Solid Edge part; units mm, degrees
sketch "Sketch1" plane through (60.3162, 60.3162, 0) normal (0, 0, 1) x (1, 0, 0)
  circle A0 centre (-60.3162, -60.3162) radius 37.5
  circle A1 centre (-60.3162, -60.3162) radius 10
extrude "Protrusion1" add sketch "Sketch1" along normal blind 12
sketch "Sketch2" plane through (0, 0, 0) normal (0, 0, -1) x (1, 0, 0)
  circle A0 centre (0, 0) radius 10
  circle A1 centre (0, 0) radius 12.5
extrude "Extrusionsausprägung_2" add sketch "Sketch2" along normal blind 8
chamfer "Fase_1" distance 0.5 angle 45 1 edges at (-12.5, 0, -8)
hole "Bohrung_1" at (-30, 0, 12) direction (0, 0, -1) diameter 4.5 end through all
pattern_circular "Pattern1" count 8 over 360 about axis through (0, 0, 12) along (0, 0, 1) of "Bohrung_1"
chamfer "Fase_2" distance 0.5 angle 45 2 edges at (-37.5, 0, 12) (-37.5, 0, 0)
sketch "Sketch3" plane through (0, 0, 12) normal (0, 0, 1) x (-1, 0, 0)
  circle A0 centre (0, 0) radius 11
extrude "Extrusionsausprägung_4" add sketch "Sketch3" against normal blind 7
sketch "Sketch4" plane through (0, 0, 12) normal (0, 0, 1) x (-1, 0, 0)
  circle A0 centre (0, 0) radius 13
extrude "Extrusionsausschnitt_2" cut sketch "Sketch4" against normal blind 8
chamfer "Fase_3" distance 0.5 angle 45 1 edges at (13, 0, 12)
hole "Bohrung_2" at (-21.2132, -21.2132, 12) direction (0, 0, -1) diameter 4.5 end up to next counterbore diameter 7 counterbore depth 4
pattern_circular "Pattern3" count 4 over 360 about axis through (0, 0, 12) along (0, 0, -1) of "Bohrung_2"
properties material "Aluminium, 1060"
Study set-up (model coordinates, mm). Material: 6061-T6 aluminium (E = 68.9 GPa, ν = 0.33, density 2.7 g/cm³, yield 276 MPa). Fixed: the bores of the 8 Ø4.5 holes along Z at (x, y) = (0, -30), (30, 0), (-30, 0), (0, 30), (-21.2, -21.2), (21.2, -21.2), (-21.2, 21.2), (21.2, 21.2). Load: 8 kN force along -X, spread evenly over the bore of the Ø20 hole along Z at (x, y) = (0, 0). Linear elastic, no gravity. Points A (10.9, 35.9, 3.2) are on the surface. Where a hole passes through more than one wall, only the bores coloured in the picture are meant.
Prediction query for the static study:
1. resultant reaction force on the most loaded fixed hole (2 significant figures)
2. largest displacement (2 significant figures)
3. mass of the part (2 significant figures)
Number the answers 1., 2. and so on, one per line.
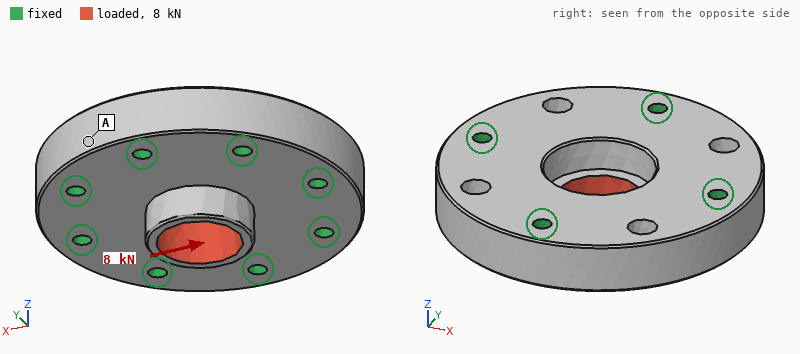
1. 1.8 kN
2. 27 µm
3. 130 g
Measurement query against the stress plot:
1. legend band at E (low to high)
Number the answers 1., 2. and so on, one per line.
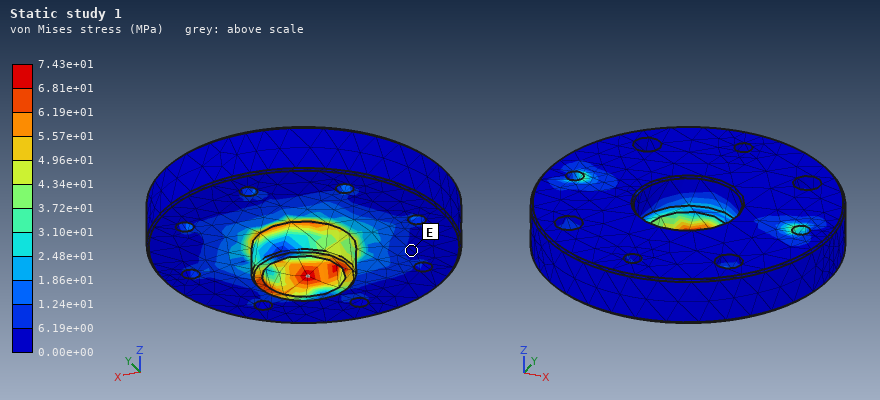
1. 0.00e+00 to 6.19e+00 MPa
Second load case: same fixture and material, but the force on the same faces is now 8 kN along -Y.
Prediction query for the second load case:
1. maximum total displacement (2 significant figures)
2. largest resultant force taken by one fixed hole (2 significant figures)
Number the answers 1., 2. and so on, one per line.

1. 26 µm
2. 1.8 kN
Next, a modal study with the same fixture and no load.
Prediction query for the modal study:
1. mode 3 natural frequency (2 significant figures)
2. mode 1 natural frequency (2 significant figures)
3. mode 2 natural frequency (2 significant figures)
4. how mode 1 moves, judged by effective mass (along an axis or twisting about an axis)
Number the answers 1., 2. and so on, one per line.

1. 31 kHz
2. 24 kHz
3. 31 kHz
4. along Z
